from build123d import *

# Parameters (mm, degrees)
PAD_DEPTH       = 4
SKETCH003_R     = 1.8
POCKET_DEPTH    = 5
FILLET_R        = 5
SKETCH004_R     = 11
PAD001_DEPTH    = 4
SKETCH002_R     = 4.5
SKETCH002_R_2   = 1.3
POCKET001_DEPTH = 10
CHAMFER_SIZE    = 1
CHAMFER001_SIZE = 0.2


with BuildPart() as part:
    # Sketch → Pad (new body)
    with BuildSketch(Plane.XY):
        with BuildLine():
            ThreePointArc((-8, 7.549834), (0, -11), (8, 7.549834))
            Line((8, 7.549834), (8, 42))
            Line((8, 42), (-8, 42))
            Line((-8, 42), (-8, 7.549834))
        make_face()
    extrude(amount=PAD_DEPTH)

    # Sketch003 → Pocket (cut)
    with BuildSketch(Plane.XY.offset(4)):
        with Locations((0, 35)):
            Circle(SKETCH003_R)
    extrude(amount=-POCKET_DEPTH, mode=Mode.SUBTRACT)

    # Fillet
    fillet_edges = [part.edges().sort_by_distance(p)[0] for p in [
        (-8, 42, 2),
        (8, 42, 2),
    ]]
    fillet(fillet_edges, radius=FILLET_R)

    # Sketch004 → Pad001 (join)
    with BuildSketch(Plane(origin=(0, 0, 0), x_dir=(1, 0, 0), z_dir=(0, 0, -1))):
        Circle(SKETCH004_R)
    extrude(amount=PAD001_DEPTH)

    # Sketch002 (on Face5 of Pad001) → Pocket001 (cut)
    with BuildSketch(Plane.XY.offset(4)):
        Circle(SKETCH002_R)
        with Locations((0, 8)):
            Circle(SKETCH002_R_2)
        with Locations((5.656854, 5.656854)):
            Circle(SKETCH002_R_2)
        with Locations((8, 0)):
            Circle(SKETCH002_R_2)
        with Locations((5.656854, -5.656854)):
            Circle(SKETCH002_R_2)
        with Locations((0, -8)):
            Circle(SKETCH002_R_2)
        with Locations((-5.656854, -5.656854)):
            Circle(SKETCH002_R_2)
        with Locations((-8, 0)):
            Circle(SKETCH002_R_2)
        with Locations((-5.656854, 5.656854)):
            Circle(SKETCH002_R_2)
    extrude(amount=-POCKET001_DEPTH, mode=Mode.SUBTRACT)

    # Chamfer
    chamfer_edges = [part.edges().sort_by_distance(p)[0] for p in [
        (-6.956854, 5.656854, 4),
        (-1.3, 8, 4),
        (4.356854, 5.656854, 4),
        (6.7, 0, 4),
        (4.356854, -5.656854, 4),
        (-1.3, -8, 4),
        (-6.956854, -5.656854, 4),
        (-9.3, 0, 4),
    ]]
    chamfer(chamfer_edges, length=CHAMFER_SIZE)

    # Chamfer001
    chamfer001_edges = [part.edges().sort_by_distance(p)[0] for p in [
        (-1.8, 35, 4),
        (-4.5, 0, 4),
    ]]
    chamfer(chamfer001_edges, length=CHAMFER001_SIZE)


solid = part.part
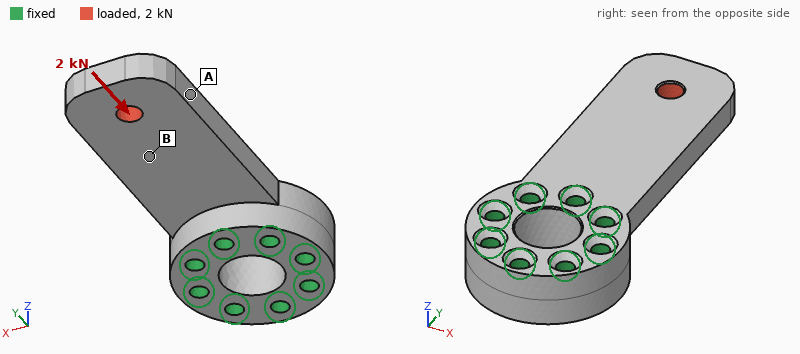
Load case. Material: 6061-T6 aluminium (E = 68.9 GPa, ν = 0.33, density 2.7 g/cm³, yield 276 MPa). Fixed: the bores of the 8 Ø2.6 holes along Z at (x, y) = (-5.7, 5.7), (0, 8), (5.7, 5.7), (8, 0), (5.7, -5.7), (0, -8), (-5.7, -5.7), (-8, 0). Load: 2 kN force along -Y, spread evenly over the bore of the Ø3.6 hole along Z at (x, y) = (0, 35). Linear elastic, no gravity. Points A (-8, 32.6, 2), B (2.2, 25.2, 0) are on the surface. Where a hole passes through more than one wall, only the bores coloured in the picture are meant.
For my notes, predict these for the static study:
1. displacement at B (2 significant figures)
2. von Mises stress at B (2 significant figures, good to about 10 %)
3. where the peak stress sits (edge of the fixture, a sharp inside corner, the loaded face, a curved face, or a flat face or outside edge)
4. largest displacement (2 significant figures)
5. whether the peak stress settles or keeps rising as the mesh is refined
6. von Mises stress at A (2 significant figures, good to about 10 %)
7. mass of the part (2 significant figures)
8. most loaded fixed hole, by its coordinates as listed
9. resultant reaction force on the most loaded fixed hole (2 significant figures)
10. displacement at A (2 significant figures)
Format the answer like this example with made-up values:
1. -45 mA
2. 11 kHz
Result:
1. 8.8 µm
2. 39 MPa
3. edge of the fixture
4. 18 µm
5. keeps rising
6. 12 MPa
7. 11 g
8. (0, 8)
9. 820 N
10. 11 µm
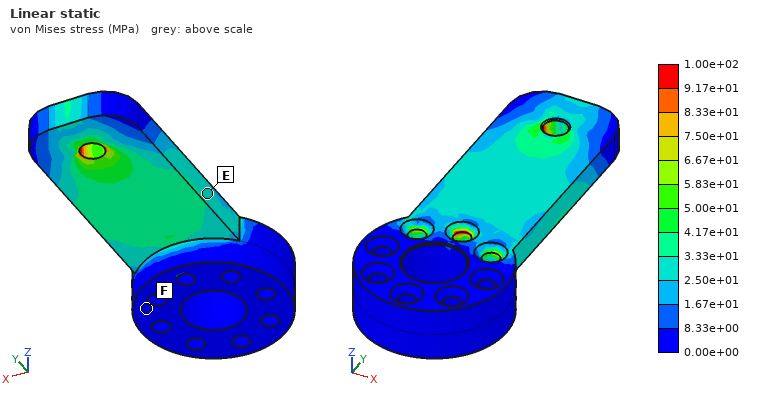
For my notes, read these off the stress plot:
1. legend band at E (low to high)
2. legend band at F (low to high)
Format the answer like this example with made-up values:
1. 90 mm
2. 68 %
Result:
1. 2.50e+01 to 3.33e+01 MPa
2. 0.00e+00 to 8.33e+00 MPa
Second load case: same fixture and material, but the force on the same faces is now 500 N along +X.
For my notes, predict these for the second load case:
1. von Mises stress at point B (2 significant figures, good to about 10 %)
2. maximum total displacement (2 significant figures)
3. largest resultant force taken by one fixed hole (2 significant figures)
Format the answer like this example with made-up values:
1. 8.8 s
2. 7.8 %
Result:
1. 22 MPa
2. 67 µm
3. 960 N
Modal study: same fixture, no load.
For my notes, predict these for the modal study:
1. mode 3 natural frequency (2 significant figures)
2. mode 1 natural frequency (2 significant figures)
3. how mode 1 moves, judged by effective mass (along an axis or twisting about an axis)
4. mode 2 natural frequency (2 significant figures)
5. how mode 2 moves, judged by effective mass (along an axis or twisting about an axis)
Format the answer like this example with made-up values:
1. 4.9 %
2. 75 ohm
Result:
1. 12 kHz
2. 3100 Hz
3. along Z
4. 9600 Hz
5. along X
